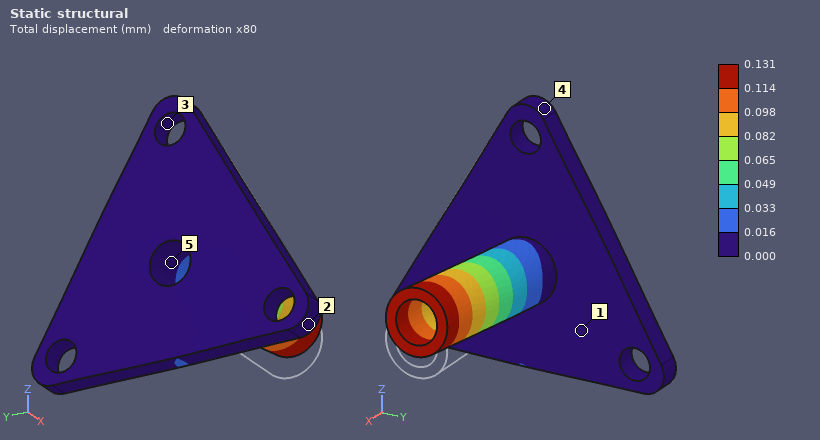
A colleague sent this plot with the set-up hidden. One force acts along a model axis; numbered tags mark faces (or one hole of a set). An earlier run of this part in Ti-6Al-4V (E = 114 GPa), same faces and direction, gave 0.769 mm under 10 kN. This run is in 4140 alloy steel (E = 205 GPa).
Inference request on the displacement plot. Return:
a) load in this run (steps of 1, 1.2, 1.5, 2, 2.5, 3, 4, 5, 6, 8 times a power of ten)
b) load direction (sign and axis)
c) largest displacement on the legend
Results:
3 kN
+Z
0.131 mm
